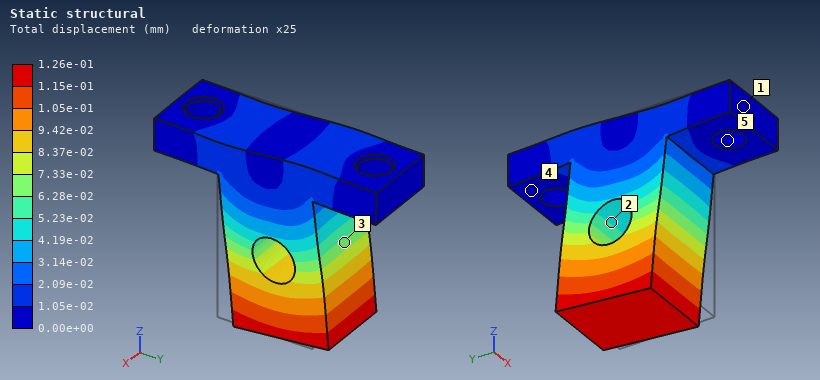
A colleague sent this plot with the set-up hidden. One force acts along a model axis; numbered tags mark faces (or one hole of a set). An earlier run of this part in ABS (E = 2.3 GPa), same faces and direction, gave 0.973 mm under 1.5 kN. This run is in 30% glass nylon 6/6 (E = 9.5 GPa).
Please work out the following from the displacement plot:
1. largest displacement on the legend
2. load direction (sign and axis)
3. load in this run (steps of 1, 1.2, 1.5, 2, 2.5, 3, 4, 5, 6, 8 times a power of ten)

1.26e-01 mm
+Y
800 N
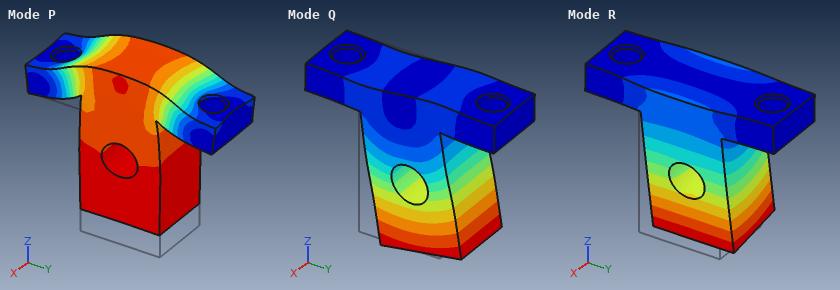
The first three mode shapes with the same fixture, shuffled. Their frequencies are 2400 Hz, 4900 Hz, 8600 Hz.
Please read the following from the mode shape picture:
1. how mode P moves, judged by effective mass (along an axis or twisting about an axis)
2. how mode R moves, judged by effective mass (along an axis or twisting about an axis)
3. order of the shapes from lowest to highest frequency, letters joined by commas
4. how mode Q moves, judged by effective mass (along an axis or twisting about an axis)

along Z
along X
R, Q, P
along Y
